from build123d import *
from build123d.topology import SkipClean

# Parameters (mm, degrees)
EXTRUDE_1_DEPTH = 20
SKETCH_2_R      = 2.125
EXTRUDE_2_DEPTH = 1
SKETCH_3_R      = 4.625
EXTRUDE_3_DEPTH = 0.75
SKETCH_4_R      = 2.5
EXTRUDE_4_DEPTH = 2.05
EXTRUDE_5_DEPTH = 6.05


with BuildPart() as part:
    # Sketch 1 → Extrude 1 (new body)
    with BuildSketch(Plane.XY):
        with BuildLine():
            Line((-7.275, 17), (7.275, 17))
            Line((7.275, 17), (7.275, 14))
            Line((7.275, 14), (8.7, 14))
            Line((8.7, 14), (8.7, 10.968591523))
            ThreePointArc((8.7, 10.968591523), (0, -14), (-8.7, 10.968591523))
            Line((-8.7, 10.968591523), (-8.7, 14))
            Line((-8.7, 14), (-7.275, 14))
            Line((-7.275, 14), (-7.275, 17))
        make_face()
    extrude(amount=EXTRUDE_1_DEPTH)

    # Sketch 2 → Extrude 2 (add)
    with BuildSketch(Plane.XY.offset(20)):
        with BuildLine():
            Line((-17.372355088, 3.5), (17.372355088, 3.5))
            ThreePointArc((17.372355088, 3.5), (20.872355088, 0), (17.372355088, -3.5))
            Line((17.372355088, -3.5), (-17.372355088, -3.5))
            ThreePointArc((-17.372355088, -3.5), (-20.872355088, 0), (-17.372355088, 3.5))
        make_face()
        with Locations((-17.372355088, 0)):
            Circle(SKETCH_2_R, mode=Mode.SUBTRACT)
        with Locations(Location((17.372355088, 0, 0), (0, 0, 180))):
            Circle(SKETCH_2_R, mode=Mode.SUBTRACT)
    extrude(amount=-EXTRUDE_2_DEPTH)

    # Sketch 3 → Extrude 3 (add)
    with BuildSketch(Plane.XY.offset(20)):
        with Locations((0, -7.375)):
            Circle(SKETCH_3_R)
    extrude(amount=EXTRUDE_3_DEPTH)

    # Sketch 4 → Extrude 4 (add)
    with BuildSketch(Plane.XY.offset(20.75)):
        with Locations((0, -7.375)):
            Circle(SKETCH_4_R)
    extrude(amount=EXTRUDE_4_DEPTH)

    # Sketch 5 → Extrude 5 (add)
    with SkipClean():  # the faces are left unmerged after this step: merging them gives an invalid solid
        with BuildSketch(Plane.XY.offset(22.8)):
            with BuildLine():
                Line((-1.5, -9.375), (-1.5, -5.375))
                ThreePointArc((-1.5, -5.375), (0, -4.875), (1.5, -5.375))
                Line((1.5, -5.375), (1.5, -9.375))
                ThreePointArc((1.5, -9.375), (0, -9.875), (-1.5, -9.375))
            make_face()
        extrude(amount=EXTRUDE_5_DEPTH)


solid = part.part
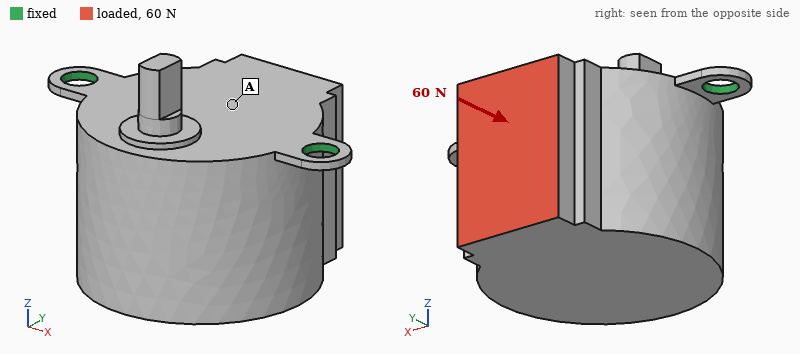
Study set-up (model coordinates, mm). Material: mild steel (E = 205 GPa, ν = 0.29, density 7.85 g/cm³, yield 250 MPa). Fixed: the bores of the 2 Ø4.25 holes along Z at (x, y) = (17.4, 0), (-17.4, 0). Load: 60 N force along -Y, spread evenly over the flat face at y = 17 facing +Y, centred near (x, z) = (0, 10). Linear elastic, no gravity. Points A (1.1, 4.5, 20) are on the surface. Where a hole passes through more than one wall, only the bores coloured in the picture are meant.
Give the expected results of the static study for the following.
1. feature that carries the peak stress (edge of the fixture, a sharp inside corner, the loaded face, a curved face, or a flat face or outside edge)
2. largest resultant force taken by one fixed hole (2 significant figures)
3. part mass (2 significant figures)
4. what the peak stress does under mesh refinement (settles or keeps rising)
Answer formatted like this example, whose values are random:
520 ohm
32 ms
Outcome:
edge of the fixture
30 N
110 g
keeps rising
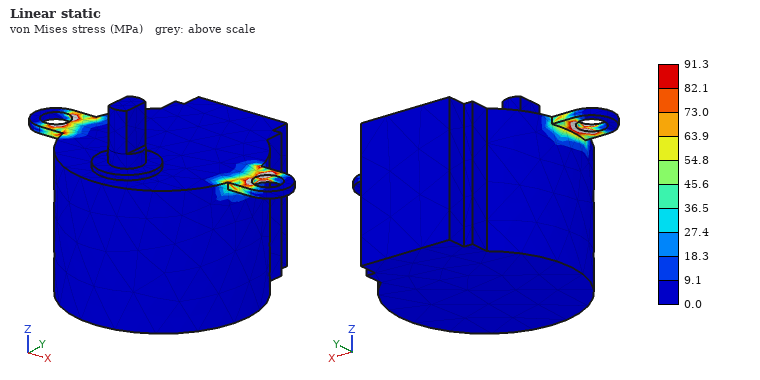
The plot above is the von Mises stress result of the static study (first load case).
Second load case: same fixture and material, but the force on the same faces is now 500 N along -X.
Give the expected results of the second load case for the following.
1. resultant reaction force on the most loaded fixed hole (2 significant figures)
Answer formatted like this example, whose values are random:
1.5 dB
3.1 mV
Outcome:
410 N
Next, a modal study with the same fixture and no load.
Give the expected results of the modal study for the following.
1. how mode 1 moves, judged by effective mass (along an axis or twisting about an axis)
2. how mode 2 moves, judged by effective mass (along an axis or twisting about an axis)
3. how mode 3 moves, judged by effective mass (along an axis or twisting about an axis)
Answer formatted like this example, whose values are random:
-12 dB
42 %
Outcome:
along Y
along Z
along X
